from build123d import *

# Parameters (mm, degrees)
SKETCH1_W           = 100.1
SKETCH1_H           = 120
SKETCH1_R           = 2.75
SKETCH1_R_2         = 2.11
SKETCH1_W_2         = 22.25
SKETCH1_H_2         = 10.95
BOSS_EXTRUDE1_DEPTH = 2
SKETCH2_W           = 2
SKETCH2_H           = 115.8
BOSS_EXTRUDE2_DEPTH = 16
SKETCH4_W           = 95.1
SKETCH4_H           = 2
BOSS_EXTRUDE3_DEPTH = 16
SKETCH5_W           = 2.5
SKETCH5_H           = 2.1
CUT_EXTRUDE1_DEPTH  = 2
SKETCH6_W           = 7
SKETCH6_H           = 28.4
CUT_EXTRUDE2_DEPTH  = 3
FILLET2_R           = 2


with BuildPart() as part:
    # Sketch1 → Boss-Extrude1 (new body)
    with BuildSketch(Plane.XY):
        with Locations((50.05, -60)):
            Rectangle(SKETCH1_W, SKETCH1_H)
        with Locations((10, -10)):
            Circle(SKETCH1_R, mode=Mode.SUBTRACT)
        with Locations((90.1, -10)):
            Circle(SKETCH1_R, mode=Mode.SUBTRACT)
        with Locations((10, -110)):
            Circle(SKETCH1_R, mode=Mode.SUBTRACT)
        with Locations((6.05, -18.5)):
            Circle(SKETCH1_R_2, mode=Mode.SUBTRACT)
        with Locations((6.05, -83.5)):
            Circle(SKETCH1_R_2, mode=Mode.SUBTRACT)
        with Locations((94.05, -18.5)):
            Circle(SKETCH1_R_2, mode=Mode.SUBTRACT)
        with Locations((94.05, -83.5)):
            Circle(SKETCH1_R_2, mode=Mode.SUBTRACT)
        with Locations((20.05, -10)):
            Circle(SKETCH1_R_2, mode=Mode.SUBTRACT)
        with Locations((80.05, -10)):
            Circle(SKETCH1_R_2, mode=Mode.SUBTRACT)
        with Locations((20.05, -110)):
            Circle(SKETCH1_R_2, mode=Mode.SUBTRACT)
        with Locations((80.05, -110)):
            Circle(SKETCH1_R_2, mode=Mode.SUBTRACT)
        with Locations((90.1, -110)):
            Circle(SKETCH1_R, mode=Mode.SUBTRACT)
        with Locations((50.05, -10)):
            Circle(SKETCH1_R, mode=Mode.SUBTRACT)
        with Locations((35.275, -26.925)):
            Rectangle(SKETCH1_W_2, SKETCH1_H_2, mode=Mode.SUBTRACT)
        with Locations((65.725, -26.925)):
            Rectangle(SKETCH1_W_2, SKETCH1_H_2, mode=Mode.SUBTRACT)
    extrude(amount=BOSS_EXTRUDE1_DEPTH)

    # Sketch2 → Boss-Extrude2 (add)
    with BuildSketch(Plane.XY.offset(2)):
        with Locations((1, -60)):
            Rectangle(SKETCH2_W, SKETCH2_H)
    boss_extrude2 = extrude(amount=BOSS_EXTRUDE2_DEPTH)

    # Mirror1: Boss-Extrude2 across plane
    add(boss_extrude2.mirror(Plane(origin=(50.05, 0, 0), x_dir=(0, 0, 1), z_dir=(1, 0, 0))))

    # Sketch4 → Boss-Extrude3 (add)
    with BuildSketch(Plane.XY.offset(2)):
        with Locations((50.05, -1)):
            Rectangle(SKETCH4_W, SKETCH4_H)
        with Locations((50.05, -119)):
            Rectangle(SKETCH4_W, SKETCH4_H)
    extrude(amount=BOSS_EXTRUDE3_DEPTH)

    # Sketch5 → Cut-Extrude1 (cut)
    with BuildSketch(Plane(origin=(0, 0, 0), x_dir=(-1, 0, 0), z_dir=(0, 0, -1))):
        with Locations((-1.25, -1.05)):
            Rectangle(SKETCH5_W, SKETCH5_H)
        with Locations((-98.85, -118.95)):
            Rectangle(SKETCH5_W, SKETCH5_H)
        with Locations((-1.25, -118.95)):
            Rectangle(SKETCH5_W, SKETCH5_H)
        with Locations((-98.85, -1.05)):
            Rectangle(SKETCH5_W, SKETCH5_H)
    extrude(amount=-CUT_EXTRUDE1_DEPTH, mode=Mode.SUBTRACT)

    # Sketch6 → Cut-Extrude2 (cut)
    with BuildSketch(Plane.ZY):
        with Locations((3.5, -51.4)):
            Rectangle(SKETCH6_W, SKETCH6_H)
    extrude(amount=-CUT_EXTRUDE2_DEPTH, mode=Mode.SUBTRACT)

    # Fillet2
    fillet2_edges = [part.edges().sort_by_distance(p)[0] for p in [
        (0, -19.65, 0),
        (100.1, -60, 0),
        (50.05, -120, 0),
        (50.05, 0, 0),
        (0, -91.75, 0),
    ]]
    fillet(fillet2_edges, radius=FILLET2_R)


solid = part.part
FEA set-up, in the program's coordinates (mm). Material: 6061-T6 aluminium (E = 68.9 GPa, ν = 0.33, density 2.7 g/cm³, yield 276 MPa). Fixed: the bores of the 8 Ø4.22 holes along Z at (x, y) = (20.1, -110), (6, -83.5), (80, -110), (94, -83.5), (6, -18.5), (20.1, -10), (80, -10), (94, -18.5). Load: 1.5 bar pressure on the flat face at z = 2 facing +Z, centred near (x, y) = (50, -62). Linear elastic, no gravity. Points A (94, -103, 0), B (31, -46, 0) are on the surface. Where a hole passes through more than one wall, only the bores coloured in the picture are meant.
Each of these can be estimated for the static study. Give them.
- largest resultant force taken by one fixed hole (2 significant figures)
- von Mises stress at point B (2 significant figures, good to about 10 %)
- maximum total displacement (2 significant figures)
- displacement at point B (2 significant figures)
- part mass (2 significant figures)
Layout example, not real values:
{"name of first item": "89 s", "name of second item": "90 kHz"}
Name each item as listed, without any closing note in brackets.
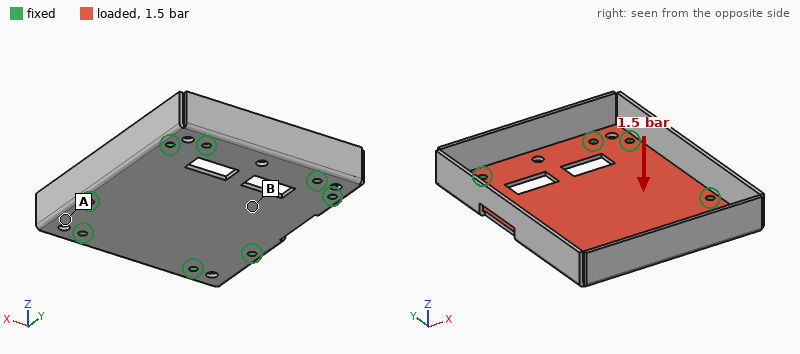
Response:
{"largest resultant force taken by one fixed hole": "280 N", "von Mises stress at point B": "45 MPa", "maximum total displacement": "0.53 mm", "displacement at point B": "0.40 mm", "part mass": "95 g"}
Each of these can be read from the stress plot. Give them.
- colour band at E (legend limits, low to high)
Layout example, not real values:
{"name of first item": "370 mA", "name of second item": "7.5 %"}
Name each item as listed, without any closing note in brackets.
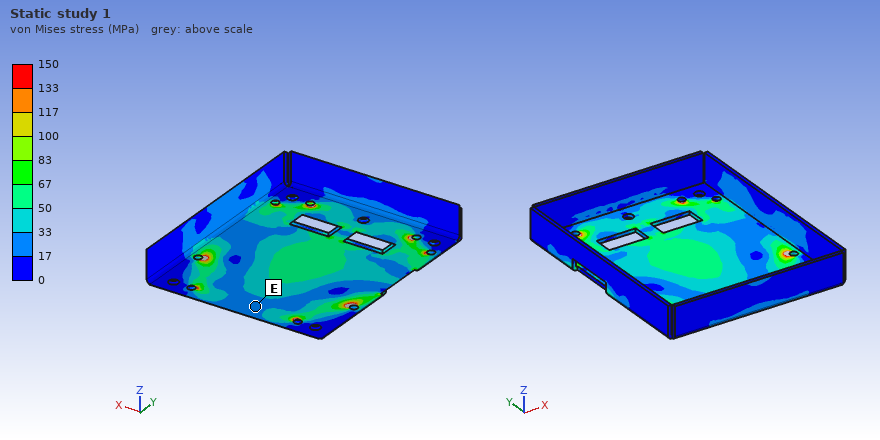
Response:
{"colour band at E": "17 to 33 MPa"}
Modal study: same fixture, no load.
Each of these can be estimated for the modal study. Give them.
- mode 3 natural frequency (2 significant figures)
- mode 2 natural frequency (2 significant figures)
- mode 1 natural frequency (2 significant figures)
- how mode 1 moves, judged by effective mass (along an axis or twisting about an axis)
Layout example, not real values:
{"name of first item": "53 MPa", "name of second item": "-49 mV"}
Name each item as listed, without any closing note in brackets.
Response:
{"mode 3 natural frequency": "2800 Hz", "mode 2 natural frequency": "2600 Hz", "mode 1 natural frequency": "1400 Hz", "how mode 1 moves, judged by effective mass": "along Z"}
